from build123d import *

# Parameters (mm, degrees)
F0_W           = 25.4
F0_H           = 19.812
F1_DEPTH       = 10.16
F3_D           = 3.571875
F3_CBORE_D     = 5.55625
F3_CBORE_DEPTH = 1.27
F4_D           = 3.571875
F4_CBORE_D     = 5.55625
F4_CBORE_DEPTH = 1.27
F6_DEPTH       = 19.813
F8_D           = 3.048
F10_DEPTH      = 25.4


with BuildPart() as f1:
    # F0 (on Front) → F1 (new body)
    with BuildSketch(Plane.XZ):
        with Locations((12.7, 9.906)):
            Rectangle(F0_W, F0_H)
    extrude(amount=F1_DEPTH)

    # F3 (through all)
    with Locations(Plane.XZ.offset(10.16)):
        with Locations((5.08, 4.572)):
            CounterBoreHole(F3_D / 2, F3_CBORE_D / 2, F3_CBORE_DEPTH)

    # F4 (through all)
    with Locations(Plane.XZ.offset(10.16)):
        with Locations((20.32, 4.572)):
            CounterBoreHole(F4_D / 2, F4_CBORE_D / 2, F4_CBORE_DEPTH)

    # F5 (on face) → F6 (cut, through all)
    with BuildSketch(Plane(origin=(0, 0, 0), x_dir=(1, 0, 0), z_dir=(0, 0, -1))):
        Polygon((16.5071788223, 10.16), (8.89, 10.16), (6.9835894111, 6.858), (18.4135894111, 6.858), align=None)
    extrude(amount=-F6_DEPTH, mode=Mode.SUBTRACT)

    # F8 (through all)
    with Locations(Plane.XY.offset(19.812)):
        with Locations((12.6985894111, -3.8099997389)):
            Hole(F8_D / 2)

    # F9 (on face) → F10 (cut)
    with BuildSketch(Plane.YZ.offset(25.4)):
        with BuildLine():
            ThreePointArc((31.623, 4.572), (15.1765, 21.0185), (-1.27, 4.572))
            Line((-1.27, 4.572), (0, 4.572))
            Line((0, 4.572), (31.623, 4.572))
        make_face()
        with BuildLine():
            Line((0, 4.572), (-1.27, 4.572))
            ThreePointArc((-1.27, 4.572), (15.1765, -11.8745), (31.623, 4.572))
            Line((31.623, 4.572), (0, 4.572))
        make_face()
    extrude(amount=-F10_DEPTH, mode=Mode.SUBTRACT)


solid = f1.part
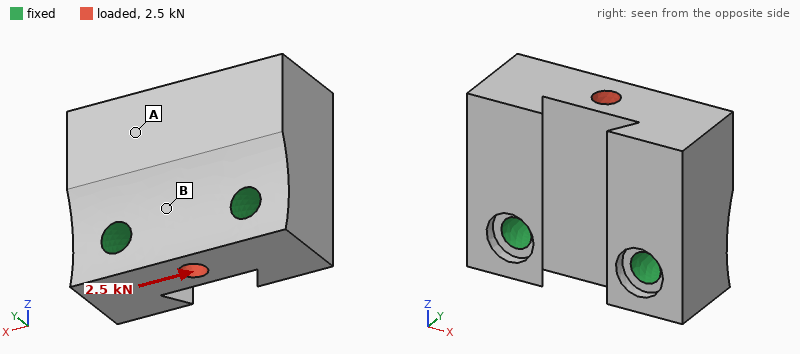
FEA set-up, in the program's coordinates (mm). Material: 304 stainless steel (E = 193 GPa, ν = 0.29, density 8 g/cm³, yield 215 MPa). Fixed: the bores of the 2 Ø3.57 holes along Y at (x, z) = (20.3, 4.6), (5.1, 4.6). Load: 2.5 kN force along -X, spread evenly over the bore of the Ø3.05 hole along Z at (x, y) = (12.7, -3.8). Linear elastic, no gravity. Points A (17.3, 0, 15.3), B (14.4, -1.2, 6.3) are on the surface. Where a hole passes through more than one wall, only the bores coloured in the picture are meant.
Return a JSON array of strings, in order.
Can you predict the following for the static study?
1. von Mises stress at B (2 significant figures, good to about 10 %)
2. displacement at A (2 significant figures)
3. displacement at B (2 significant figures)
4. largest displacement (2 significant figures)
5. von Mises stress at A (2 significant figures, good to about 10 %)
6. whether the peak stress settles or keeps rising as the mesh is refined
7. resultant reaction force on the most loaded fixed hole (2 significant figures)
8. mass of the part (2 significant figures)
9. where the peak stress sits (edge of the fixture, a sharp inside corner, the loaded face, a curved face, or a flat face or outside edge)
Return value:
["18 MPa", "1.7 µm", "0.61 µm", "2.3 µm", "6.4 MPa", "keeps rising", "1.4 kN", "31 g", "edge of the fixture"]
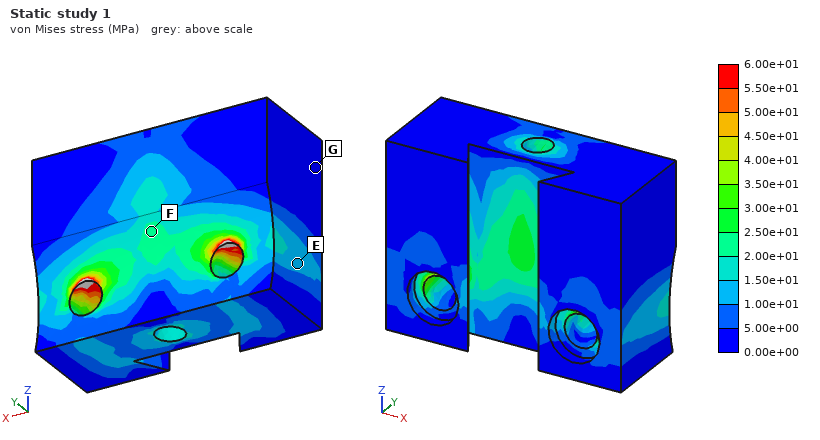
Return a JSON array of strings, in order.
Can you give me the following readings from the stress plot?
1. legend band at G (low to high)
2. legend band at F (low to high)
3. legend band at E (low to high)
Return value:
["0.00e+00 to 5.00e+00 MPa", "2.00e+01 to 2.50e+01 MPa", "1.00e+01 to 1.50e+01 MPa"]
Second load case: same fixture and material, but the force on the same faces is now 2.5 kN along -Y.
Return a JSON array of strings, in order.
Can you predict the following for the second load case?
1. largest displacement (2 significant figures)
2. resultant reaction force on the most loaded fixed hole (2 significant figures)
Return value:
["7.9 µm", "1.3 kN"]
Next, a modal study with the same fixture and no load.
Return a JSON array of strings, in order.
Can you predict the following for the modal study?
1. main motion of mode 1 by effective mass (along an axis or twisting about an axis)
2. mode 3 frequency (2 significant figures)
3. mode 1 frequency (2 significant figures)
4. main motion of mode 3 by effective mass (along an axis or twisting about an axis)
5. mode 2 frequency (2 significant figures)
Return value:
["along Y", "34 kHz", "21 kHz", "along X", "28 kHz"]
